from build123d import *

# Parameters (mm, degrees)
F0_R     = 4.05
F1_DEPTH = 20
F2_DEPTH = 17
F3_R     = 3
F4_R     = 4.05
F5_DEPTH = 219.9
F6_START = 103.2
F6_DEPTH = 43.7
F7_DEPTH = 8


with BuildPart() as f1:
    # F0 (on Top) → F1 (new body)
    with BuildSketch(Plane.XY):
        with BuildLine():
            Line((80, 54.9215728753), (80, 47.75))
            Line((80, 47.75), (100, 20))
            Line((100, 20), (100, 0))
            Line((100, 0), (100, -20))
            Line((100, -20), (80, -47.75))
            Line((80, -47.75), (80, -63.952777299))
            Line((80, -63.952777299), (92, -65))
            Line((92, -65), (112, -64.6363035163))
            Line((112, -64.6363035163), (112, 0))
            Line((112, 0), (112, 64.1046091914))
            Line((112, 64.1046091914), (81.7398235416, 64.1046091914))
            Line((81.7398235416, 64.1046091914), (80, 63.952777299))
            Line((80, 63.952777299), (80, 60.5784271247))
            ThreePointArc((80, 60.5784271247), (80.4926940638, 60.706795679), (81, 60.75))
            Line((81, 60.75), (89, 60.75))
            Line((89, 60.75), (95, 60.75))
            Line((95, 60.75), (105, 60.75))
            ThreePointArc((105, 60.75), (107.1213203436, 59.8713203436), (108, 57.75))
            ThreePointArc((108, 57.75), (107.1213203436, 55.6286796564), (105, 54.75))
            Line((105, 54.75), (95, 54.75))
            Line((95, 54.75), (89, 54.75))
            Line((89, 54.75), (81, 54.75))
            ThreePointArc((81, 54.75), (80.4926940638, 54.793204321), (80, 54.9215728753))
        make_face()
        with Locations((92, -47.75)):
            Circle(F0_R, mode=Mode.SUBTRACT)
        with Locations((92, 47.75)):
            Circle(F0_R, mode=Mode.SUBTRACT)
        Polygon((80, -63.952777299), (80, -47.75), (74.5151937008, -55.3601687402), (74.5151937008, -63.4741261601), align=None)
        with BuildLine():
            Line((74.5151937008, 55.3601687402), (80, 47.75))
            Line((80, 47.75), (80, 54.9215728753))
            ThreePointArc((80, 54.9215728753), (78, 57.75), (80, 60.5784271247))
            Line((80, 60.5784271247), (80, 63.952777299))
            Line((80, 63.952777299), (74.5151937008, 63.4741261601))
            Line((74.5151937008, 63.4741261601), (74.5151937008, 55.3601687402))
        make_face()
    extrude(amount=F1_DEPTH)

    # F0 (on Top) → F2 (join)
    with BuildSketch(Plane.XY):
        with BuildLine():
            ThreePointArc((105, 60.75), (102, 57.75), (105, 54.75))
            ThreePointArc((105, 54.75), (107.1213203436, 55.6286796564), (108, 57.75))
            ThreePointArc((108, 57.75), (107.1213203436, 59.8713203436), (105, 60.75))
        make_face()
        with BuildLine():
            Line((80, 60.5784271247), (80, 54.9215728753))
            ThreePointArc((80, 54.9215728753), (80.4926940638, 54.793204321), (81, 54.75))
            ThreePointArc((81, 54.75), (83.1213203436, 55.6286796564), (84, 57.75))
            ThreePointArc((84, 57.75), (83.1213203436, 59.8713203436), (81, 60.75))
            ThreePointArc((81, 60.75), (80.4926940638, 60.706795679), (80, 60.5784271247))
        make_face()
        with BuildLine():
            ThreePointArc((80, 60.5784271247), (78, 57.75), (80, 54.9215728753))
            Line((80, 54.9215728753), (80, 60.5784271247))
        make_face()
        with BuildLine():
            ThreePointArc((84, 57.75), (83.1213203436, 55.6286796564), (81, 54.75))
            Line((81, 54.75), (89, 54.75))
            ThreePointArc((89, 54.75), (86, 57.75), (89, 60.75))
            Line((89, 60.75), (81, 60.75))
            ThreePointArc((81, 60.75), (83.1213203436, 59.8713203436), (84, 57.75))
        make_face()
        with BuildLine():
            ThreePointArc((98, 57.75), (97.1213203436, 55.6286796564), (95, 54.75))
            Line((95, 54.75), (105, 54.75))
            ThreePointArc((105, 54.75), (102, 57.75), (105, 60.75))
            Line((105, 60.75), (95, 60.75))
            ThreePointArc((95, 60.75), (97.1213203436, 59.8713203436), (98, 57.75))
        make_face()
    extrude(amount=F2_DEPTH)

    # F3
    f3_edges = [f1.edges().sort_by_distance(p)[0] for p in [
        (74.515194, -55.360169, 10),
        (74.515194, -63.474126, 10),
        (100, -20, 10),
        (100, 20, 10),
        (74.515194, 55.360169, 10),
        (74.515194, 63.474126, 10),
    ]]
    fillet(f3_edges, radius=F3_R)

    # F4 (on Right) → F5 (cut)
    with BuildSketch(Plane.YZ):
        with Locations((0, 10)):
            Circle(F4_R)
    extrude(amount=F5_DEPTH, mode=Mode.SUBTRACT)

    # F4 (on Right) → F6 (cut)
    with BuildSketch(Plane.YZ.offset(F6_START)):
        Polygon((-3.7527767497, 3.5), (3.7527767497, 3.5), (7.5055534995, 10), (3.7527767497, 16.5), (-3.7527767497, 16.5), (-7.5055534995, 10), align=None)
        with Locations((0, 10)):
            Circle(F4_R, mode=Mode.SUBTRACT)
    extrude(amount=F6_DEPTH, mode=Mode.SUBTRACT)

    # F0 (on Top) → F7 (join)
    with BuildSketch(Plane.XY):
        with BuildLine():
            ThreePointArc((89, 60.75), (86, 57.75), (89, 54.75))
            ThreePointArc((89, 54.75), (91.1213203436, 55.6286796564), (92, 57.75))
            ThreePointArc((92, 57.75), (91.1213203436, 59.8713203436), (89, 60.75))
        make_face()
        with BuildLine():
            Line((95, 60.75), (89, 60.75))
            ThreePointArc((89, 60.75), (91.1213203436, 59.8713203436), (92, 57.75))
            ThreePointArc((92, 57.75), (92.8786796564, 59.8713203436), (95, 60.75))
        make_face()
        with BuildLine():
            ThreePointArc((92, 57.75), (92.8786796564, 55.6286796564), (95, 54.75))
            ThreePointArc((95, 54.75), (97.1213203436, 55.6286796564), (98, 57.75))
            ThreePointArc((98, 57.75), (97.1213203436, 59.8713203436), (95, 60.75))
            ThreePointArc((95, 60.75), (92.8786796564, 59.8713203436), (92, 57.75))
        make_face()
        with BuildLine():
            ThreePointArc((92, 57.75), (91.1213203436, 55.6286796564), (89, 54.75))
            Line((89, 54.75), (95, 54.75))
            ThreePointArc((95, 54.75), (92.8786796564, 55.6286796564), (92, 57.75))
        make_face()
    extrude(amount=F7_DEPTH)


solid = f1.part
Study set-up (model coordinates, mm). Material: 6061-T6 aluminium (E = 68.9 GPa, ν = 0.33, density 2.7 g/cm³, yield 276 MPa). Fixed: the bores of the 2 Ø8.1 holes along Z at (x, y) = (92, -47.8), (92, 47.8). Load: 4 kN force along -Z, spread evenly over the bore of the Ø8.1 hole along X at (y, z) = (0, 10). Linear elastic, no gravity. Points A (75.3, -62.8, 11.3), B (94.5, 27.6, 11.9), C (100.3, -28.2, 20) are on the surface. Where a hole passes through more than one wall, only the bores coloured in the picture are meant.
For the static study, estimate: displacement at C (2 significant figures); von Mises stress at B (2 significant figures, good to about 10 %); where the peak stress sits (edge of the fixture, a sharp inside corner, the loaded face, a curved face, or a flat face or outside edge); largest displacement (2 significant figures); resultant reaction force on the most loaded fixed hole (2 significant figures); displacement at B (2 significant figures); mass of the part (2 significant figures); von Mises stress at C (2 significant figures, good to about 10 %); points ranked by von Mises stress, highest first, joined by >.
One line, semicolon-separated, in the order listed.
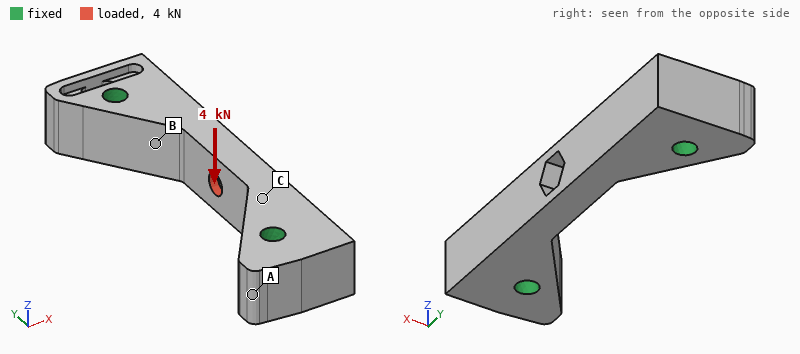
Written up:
16 µm; 29 MPa; a sharp inside corner; 53 µm; 2.0 kN; 12 µm; 140 g; 17 MPa; B > C > A
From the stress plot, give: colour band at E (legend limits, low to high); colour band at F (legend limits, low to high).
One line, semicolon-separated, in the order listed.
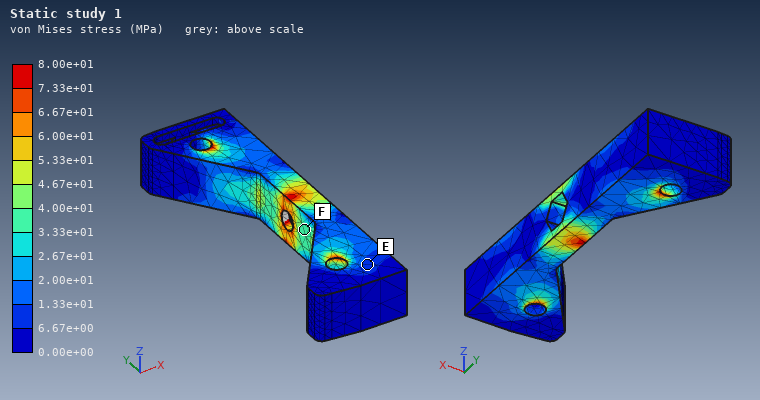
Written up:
6.67e+00 to 1.33e+01 MPa; 3.33e+01 to 4.00e+01 MPa
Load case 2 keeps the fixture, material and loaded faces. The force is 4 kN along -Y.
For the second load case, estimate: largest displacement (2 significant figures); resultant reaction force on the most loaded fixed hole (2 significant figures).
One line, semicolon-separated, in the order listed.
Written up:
14 µm; 2.0 kN
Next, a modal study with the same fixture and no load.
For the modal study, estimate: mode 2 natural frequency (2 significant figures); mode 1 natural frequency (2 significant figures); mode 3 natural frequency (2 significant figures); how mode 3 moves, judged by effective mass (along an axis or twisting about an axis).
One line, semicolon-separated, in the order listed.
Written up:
10 kHz; 10 kHz; 13 kHz; along Y
